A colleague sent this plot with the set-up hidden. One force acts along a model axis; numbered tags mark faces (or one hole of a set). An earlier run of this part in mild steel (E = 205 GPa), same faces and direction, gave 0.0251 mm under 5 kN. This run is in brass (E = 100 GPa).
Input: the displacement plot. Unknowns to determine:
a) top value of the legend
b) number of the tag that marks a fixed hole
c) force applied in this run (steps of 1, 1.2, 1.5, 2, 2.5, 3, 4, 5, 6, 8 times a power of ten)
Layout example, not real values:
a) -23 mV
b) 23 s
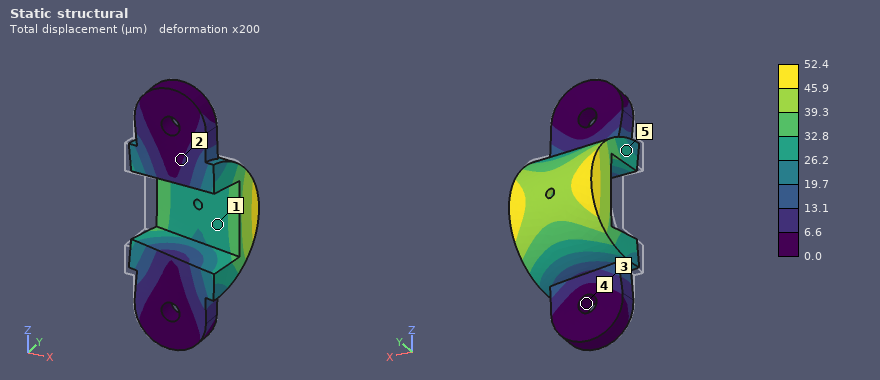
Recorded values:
a) 52.4 µm
b) 4
c) 5 kN
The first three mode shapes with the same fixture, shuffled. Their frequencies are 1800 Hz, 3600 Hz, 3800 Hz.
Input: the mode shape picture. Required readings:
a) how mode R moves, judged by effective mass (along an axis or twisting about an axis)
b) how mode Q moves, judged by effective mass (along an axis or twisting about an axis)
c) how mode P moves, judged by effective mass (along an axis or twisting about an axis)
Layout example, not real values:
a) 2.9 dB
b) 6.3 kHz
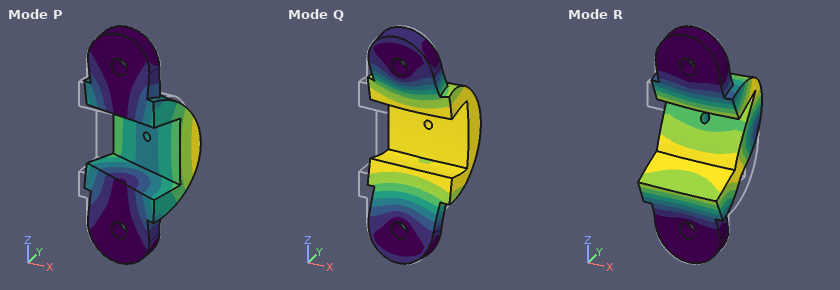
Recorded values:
a) along Z
b) along Y
c) along X
